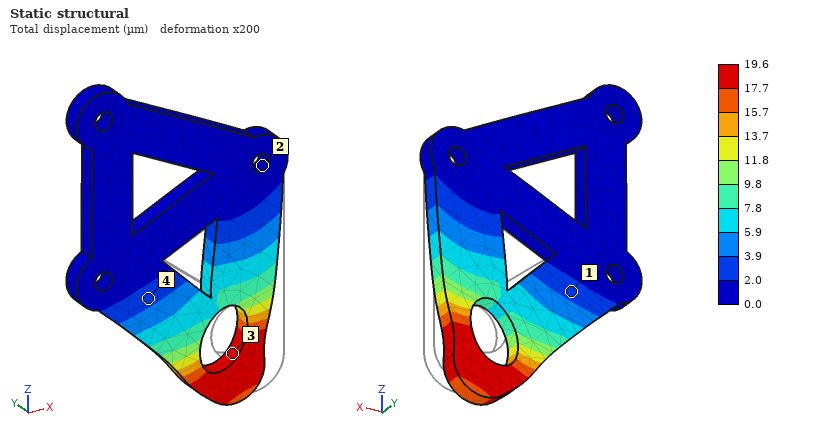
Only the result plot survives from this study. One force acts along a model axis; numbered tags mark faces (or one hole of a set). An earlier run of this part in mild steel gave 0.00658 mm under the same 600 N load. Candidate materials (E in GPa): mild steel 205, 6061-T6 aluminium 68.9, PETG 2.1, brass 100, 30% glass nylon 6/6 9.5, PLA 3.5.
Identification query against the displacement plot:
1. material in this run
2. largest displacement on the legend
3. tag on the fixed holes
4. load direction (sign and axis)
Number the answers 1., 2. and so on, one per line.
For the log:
1. 6061-T6 aluminium
2. 19.6 µm
3. 2
4. -X
